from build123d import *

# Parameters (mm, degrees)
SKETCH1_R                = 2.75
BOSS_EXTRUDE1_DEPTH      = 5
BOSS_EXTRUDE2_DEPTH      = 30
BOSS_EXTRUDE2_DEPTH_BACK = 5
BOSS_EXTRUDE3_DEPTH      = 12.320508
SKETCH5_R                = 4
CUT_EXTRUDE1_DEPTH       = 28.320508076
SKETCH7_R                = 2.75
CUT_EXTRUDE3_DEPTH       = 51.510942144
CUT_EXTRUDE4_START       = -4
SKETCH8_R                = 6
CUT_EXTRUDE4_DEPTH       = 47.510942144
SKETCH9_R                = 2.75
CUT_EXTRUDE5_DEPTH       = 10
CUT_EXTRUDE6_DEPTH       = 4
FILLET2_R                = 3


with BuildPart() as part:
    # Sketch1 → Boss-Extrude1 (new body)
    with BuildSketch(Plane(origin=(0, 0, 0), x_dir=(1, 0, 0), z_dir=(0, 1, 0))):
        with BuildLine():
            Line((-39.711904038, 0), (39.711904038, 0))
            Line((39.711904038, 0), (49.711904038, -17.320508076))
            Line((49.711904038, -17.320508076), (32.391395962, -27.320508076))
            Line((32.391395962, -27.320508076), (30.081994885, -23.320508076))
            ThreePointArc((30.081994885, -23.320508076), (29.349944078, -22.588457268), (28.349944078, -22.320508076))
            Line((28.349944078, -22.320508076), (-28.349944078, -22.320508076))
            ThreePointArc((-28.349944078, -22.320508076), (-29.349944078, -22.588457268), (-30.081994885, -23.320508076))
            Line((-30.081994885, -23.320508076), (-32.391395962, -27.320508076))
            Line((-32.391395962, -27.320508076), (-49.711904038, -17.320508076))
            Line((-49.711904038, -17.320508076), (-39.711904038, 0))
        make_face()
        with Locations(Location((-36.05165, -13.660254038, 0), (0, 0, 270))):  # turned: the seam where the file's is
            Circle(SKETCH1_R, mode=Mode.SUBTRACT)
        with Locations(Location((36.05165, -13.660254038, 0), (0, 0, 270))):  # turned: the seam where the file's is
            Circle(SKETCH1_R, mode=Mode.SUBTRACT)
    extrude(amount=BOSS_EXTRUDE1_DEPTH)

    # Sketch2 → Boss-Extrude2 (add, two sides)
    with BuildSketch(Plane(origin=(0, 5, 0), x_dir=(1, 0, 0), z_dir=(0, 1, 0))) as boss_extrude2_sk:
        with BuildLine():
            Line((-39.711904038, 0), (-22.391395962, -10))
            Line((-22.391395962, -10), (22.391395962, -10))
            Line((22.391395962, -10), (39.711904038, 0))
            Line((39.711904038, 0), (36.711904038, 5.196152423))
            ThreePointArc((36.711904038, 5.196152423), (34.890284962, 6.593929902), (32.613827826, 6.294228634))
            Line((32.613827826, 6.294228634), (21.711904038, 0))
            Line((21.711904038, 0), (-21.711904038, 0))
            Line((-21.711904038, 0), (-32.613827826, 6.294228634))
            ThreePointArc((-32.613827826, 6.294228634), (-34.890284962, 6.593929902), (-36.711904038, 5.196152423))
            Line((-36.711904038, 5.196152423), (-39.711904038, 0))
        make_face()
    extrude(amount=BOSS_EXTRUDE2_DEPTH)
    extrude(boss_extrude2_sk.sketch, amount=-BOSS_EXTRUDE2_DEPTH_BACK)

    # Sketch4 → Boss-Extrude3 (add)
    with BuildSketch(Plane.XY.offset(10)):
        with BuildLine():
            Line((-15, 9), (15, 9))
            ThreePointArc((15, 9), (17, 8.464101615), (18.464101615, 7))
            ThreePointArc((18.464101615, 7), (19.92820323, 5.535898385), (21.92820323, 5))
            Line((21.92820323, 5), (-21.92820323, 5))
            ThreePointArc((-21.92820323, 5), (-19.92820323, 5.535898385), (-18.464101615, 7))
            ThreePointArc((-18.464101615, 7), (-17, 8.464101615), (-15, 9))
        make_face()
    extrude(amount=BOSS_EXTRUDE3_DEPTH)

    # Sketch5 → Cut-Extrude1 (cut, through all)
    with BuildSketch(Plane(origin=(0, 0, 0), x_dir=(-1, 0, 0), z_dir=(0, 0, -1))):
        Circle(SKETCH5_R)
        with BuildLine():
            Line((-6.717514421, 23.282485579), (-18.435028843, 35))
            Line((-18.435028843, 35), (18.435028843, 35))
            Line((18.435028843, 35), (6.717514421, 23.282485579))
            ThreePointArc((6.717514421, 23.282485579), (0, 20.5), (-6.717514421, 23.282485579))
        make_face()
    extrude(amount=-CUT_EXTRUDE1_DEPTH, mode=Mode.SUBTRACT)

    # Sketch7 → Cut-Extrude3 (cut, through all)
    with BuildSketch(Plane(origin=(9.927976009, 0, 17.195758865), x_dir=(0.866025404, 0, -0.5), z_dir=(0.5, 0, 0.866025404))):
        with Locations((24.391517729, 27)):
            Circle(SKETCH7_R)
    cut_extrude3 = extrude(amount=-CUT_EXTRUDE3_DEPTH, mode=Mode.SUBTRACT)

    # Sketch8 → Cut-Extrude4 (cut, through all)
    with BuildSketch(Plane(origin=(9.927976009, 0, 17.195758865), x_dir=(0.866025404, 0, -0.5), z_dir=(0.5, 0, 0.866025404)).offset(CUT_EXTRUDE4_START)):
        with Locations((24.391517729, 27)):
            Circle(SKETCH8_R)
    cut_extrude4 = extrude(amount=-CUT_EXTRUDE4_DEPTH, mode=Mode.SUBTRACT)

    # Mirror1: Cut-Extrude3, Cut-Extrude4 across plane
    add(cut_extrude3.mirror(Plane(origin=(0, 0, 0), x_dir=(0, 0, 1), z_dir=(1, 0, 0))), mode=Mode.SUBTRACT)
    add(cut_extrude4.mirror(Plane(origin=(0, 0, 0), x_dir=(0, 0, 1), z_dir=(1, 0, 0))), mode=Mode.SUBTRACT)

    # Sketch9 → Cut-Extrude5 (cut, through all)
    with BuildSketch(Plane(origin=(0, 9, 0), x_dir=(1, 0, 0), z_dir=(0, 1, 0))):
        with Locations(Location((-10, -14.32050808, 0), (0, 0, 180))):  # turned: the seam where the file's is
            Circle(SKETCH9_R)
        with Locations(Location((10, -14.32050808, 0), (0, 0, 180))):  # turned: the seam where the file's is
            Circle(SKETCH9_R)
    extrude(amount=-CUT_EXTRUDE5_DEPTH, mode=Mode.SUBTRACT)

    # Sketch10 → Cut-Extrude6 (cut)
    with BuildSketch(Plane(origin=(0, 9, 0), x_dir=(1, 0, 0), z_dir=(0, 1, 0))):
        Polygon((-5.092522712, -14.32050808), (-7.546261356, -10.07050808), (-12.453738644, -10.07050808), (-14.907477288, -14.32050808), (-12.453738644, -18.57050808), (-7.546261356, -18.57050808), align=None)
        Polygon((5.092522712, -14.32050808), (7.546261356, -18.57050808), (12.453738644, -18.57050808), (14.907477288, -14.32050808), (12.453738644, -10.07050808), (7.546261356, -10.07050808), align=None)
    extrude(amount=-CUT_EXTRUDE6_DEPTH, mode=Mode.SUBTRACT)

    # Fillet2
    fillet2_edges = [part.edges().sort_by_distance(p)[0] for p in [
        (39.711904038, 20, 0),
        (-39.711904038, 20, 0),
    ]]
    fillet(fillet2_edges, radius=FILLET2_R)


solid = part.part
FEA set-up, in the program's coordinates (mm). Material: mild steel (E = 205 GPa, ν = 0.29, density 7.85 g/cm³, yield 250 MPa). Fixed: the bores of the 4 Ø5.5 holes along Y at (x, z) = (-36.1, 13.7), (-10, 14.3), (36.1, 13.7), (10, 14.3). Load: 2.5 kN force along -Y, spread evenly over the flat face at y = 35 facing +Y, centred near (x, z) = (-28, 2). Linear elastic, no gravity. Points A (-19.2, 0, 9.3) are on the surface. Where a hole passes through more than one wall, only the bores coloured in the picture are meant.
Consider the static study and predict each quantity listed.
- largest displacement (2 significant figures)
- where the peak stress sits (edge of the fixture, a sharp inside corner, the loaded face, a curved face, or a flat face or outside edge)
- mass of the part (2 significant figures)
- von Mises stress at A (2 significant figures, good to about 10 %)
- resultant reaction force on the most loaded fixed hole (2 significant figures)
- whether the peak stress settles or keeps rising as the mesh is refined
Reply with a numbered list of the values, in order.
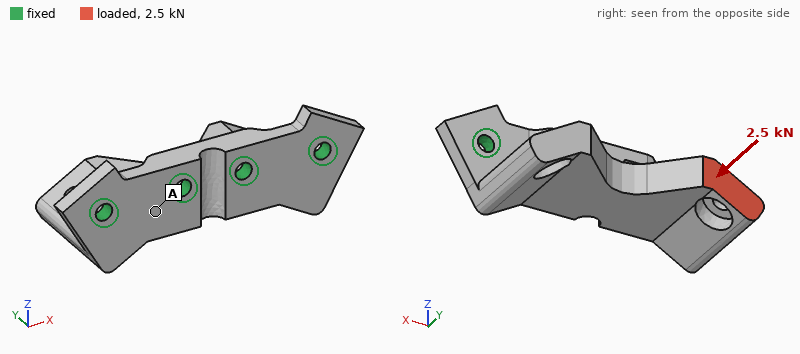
1. 39 µm
2. edge of the fixture
3. 230 g
4. 29 MPa
5. 1.4 kN
6. keeps rising
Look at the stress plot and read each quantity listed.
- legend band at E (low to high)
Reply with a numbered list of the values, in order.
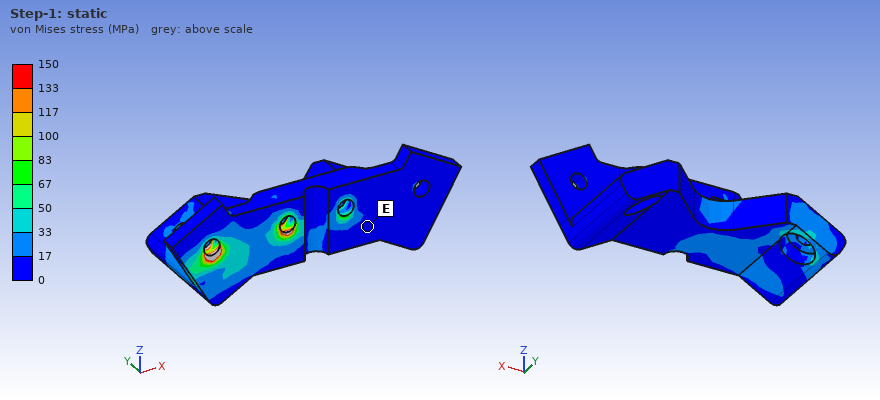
1. 0 to 17 MPa
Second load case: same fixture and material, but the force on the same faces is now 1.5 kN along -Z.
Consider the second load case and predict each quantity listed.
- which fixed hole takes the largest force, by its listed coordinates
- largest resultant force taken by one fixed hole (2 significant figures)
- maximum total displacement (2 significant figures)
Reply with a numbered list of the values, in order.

1. (-10, 14.3)
2. 1.2 kN
3. 0.10 mm
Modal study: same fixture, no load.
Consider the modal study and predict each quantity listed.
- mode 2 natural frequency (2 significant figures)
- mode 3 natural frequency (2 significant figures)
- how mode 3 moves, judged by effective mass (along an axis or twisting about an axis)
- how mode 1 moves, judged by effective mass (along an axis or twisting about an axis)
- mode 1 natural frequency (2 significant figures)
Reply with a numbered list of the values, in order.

1. 5900 Hz
2. 11 kHz
3. along X
4. along Z
5. 4100 Hz
